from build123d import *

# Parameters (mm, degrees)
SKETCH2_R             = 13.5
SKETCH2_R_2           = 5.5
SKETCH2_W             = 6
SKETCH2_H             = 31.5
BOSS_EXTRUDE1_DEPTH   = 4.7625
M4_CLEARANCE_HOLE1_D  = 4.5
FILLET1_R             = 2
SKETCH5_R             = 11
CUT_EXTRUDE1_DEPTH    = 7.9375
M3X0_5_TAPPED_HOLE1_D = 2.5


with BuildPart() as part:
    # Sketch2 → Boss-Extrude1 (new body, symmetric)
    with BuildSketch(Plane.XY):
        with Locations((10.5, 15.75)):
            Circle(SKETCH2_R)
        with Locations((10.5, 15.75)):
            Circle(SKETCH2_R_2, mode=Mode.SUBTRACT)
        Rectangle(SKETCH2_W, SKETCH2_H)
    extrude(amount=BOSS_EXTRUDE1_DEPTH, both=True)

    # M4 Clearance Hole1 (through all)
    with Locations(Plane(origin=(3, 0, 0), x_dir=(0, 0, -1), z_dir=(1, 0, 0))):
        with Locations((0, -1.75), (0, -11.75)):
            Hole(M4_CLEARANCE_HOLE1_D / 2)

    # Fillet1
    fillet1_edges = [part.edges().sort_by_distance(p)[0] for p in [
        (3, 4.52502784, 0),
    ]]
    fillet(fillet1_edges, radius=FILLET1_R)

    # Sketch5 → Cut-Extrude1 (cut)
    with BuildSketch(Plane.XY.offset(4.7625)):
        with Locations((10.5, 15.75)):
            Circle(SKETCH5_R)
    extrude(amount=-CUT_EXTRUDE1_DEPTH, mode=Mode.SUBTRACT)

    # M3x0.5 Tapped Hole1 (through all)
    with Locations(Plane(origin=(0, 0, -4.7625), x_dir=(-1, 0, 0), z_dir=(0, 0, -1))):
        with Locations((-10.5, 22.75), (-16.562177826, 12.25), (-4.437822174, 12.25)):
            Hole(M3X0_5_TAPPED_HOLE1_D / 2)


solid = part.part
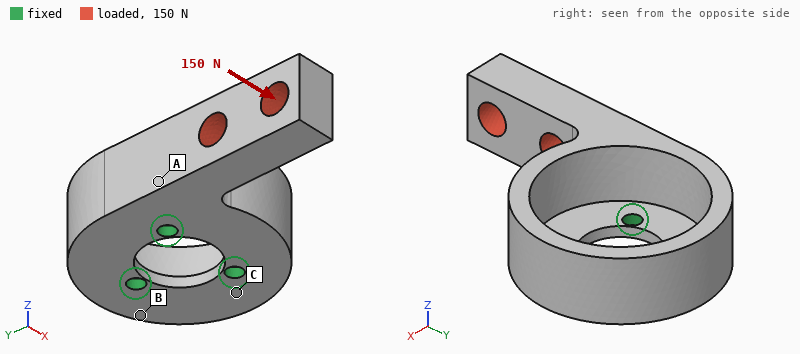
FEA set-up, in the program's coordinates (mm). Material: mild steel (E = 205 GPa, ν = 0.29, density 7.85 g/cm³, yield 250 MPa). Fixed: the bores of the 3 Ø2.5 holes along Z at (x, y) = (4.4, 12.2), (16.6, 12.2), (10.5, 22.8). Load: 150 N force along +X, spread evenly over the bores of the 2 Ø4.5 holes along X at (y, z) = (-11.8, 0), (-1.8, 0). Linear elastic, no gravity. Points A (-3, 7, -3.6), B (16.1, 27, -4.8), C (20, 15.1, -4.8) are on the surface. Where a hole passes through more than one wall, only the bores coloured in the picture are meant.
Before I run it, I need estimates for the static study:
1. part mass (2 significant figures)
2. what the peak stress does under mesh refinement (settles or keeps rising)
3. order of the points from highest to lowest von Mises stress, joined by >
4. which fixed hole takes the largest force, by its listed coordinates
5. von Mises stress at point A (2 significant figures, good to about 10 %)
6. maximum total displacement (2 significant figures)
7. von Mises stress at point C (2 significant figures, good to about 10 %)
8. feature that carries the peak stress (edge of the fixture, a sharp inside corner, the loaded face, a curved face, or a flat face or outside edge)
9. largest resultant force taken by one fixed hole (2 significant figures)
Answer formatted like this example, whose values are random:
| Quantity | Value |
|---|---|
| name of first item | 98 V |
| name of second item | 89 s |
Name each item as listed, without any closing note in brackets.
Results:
| Quantity | Value |
|---|---|
| part mass | 27 g |
| what the peak stress does under mesh refinement | keeps rising |
| order of the points from highest to lowest von Mises stress, joined by > | A > C > B |
| which fixed hole takes the largest force, by its listed coordinates | (16.6, 12.2) |
| von Mises stress at point A | 21 MPa |
| maximum total displacement | 16 µm |
| von Mises stress at point C | 10 MPa |
| feature that carries the peak stress | edge of the fixture |
| largest resultant force taken by one fixed hole | 210 N |
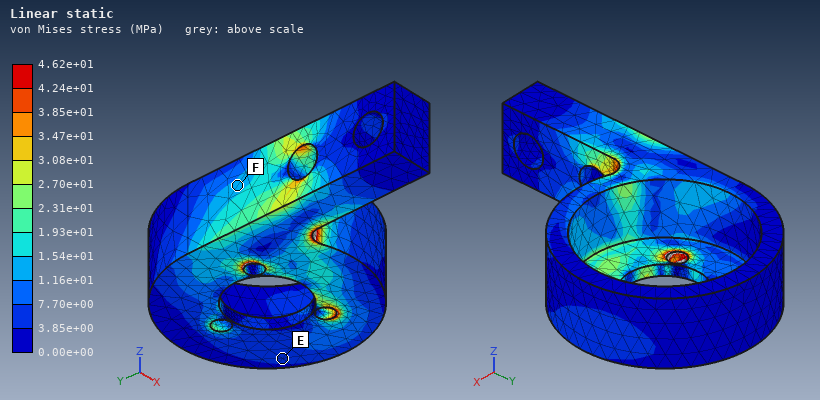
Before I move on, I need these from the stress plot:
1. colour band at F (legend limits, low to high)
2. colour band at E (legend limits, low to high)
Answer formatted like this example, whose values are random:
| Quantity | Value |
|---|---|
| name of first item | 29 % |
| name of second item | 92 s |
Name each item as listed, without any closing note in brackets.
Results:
| Quantity | Value |
|---|---|
| colour band at F | 1.16e+01 to 1.54e+01 MPa |
| colour band at E | 3.85e+00 to 7.70e+00 MPa |
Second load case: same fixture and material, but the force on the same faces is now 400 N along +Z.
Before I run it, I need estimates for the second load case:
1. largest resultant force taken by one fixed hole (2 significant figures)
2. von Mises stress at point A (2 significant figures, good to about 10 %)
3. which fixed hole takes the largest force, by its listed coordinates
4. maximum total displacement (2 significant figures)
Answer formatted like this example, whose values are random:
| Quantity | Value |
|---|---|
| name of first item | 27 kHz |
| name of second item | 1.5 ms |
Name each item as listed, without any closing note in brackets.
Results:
| Quantity | Value |
|---|---|
| largest resultant force taken by one fixed hole | 730 N |
| von Mises stress at point A | 46 MPa |
| which fixed hole takes the largest force, by its listed coordinates | (4.4, 12.2) |
| maximum total displacement | 0.10 mm |
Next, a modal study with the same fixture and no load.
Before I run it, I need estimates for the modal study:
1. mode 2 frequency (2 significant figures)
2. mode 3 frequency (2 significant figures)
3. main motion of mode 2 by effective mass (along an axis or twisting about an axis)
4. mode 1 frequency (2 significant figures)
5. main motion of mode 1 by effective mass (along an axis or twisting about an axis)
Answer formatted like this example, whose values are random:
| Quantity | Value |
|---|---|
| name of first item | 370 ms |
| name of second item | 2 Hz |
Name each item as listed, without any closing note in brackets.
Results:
| Quantity | Value |
|---|---|
| mode 2 frequency | 7500 Hz |
| mode 3 frequency | 11 kHz |
| main motion of mode 2 by effective mass | along X |
| mode 1 frequency | 4300 Hz |
| main motion of mode 1 by effective mass | along Z |
